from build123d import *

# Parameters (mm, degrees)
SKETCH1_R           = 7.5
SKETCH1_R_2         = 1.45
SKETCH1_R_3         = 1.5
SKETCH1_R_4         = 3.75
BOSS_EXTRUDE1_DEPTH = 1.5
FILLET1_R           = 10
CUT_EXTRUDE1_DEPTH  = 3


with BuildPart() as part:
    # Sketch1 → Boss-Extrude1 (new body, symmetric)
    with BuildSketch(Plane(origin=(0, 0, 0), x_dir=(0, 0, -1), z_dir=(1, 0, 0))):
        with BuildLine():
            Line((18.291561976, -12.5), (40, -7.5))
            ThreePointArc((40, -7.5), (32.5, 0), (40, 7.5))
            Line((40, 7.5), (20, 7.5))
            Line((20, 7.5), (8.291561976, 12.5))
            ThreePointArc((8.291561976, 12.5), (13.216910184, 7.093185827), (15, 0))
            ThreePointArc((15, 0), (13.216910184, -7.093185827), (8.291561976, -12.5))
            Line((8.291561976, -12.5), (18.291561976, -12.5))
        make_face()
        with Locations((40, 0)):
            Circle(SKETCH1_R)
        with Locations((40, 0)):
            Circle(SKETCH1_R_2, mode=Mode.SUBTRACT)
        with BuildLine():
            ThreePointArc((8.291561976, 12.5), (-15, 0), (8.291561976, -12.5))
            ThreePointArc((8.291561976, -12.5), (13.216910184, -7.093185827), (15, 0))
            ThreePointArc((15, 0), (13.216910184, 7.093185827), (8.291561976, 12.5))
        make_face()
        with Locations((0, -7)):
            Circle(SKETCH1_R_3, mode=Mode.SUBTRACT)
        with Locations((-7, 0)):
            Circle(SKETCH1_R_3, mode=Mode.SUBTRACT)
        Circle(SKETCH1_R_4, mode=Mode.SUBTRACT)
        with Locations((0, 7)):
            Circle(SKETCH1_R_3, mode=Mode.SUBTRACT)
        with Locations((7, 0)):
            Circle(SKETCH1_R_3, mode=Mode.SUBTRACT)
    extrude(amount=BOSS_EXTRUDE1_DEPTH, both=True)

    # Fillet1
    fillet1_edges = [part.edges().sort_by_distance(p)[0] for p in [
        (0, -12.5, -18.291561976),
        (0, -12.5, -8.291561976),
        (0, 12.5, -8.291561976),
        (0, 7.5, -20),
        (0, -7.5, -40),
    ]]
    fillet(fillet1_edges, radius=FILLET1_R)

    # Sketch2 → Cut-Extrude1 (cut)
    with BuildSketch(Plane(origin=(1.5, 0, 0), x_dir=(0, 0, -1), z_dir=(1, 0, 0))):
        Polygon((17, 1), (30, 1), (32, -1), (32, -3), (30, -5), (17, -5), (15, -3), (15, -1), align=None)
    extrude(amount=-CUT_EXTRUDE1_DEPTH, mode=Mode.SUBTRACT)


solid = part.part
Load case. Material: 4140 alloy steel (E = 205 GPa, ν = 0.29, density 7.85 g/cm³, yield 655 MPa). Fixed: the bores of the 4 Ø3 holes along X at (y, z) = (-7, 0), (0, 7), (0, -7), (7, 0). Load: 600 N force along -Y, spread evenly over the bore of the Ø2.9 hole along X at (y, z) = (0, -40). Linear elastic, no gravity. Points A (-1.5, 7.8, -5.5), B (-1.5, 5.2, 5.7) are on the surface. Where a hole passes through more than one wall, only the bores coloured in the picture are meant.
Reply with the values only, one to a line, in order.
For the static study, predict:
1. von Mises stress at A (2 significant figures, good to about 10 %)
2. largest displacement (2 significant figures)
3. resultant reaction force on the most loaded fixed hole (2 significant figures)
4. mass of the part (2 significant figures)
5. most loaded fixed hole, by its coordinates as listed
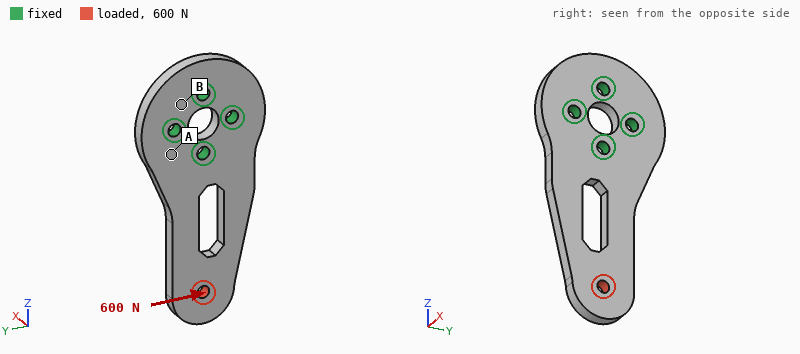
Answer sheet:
46 MPa
40 µm
1.0 kN
26 g
(-7, 0)
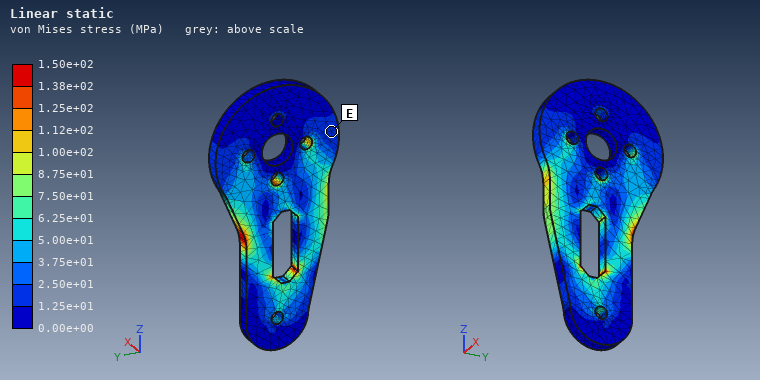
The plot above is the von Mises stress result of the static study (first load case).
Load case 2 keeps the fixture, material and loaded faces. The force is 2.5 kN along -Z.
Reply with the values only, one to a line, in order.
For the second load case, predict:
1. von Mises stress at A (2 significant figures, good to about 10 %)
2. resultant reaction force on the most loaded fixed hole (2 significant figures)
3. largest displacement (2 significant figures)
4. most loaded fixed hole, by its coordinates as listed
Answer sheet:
36 MPa
1.1 kN
13 µm
(0, -7)
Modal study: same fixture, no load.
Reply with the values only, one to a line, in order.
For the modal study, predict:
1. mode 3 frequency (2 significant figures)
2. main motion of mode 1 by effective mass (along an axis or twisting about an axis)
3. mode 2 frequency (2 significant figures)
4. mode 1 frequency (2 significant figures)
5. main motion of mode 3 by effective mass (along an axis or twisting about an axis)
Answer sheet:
8700 Hz
along X
6900 Hz
1800 Hz
along Y
